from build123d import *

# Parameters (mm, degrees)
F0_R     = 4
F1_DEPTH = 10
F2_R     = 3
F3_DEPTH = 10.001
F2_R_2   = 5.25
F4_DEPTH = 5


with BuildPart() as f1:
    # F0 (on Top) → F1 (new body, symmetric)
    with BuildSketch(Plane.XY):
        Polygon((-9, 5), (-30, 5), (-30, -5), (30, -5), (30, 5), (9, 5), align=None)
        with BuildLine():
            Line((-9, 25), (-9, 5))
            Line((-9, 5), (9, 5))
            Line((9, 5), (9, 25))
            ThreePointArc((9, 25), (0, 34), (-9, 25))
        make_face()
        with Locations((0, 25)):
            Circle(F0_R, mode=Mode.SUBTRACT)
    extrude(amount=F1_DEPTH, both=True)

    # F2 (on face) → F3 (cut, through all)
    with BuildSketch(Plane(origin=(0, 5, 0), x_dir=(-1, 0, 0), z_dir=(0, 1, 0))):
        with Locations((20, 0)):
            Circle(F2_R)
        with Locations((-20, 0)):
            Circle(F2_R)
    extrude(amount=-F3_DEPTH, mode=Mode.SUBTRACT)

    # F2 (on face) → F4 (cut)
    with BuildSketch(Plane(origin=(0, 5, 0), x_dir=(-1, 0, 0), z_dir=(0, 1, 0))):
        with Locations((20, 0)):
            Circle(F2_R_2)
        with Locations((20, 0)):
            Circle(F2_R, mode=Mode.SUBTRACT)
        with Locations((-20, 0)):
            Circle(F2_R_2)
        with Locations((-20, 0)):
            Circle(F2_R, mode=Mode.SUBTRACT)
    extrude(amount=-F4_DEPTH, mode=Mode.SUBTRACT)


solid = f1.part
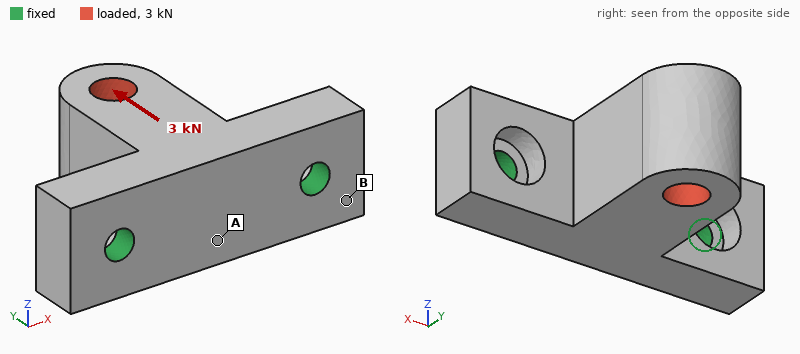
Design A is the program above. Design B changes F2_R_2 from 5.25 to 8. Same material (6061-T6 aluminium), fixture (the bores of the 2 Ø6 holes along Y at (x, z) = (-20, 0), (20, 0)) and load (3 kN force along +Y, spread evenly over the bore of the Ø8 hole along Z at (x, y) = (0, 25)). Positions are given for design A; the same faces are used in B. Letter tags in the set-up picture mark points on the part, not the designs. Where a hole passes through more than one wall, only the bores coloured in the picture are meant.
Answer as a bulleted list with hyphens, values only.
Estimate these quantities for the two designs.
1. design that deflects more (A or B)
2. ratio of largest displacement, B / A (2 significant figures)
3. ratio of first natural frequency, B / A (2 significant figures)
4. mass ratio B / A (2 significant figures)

- B
- 1.2
- 0.90
- 0.94
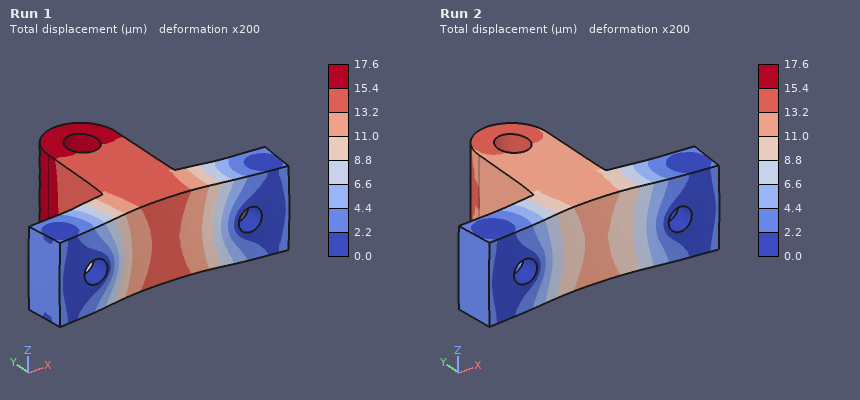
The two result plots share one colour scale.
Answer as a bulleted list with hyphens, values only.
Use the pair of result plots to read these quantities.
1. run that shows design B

- Run 1
